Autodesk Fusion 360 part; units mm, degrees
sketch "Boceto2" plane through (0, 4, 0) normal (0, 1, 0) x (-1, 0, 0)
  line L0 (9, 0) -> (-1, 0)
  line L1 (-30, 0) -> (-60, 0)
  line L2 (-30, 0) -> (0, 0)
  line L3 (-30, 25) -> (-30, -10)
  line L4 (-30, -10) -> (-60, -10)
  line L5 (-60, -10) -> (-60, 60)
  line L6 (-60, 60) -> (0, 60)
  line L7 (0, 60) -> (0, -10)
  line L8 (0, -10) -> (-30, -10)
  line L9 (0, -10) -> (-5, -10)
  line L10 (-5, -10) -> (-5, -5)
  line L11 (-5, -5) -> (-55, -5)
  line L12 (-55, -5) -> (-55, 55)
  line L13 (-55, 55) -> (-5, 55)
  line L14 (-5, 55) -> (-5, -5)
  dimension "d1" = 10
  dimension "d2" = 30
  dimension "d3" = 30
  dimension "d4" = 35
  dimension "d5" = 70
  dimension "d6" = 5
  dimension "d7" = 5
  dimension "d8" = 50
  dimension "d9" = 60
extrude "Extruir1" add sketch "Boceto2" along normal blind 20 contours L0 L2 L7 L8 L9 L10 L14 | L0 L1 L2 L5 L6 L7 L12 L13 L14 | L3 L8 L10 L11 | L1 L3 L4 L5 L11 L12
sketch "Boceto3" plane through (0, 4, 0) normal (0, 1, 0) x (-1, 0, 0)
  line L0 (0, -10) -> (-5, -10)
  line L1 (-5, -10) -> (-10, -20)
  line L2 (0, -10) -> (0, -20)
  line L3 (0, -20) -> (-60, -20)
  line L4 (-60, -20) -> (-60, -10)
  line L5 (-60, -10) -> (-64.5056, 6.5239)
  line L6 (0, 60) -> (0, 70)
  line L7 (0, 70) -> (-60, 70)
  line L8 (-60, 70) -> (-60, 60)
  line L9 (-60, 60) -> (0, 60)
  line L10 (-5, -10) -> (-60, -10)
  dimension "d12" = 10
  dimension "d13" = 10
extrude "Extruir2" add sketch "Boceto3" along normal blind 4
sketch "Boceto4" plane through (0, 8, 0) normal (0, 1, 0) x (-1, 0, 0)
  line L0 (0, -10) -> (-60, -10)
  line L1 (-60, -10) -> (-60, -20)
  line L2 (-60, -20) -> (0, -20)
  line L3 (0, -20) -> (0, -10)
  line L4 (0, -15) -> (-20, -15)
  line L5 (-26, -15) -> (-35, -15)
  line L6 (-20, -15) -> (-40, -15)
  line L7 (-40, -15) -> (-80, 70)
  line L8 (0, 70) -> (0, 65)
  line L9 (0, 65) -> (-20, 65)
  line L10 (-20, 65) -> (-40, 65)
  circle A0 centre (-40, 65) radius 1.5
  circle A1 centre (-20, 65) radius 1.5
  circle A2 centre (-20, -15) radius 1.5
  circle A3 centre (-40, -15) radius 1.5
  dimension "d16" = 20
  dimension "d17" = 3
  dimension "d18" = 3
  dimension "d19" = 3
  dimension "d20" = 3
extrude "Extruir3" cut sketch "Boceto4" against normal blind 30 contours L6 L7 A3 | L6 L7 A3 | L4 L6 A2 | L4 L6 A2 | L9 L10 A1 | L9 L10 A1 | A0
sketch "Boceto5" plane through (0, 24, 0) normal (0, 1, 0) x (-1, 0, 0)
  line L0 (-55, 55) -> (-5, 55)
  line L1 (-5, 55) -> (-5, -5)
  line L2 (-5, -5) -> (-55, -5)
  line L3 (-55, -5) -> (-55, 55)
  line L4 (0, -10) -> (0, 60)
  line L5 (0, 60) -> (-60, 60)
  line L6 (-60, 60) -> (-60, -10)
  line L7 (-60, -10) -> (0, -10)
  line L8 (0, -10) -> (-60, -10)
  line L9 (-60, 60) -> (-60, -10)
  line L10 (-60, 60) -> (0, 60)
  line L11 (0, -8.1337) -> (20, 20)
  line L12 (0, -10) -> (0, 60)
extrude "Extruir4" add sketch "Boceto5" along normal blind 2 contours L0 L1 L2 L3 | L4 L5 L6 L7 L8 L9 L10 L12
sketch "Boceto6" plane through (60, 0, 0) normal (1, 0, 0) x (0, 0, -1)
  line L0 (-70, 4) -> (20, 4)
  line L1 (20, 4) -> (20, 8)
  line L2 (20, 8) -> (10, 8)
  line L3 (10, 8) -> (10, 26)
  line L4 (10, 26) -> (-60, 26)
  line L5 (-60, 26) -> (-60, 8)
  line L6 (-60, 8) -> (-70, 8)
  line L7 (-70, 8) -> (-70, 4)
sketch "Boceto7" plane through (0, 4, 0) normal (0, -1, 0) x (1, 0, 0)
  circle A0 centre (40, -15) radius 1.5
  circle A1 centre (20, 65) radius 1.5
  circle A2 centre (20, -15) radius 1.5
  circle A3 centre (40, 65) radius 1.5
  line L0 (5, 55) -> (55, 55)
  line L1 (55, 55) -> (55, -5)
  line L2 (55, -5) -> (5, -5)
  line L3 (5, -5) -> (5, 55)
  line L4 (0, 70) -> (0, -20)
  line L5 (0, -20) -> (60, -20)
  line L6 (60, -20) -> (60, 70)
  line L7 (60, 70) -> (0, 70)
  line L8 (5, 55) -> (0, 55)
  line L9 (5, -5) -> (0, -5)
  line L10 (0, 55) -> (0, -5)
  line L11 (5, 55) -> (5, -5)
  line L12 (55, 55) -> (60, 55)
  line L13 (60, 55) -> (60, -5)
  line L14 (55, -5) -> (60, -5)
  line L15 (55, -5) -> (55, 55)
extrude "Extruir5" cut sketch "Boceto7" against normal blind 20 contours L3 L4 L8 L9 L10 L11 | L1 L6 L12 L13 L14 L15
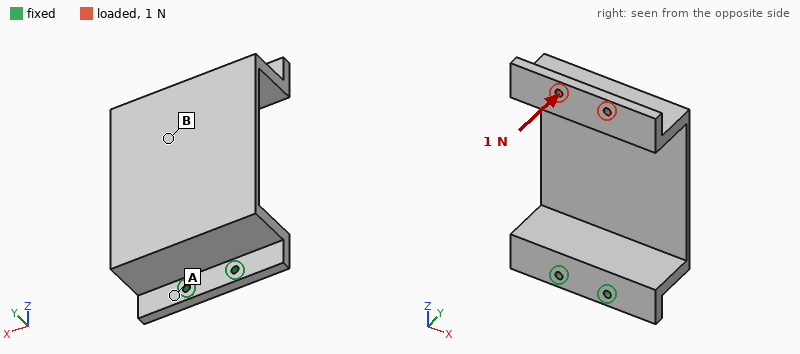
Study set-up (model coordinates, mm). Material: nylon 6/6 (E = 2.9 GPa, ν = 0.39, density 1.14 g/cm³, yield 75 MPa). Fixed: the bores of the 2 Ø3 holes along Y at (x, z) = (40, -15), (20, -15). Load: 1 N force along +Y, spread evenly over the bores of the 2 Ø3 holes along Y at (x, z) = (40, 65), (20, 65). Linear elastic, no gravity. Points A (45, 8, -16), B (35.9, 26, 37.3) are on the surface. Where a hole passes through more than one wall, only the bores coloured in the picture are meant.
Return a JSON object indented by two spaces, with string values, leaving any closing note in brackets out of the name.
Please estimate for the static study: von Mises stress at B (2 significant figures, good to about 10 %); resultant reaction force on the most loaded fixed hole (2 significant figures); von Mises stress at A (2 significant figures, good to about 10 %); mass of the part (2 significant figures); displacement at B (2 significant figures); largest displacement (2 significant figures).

{
  "von Mises stress at B": "0.61 MPa",
  "resultant reaction force on the most loaded fixed hole": "0.58 N",
  "von Mises stress at A": "0.36 MPa",
  "mass of the part": "29 g",
  "displacement at B": "0.47 mm",
  "largest displacement": "1.2 mm"
}
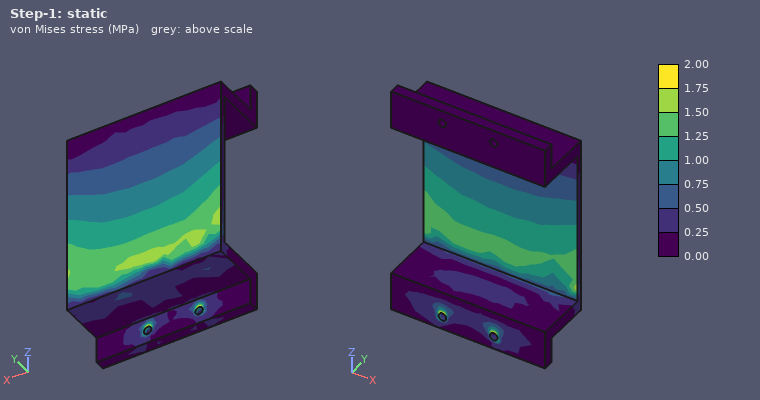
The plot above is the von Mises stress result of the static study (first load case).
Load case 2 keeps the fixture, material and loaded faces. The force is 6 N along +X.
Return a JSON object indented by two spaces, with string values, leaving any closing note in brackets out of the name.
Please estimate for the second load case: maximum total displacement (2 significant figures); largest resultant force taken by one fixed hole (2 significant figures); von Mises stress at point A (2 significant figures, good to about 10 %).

{
  "maximum total displacement": "1.1 mm",
  "largest resultant force taken by one fixed hole": "21 N",
  "von Mises stress at point A": "1.4 MPa"
}
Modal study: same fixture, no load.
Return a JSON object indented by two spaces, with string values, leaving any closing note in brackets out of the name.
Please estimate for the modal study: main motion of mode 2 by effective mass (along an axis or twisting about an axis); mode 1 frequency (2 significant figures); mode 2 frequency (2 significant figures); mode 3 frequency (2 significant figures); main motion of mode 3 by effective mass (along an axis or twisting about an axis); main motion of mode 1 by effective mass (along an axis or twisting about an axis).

{
  "main motion of mode 2 by effective mass": "along X",
  "mode 1 frequency": "50 Hz",
  "mode 2 frequency": "130 Hz",
  "mode 3 frequency": "250 Hz",
  "main motion of mode 3 by effective mass": "along Z",
  "main motion of mode 1 by effective mass": "along Y"
}
